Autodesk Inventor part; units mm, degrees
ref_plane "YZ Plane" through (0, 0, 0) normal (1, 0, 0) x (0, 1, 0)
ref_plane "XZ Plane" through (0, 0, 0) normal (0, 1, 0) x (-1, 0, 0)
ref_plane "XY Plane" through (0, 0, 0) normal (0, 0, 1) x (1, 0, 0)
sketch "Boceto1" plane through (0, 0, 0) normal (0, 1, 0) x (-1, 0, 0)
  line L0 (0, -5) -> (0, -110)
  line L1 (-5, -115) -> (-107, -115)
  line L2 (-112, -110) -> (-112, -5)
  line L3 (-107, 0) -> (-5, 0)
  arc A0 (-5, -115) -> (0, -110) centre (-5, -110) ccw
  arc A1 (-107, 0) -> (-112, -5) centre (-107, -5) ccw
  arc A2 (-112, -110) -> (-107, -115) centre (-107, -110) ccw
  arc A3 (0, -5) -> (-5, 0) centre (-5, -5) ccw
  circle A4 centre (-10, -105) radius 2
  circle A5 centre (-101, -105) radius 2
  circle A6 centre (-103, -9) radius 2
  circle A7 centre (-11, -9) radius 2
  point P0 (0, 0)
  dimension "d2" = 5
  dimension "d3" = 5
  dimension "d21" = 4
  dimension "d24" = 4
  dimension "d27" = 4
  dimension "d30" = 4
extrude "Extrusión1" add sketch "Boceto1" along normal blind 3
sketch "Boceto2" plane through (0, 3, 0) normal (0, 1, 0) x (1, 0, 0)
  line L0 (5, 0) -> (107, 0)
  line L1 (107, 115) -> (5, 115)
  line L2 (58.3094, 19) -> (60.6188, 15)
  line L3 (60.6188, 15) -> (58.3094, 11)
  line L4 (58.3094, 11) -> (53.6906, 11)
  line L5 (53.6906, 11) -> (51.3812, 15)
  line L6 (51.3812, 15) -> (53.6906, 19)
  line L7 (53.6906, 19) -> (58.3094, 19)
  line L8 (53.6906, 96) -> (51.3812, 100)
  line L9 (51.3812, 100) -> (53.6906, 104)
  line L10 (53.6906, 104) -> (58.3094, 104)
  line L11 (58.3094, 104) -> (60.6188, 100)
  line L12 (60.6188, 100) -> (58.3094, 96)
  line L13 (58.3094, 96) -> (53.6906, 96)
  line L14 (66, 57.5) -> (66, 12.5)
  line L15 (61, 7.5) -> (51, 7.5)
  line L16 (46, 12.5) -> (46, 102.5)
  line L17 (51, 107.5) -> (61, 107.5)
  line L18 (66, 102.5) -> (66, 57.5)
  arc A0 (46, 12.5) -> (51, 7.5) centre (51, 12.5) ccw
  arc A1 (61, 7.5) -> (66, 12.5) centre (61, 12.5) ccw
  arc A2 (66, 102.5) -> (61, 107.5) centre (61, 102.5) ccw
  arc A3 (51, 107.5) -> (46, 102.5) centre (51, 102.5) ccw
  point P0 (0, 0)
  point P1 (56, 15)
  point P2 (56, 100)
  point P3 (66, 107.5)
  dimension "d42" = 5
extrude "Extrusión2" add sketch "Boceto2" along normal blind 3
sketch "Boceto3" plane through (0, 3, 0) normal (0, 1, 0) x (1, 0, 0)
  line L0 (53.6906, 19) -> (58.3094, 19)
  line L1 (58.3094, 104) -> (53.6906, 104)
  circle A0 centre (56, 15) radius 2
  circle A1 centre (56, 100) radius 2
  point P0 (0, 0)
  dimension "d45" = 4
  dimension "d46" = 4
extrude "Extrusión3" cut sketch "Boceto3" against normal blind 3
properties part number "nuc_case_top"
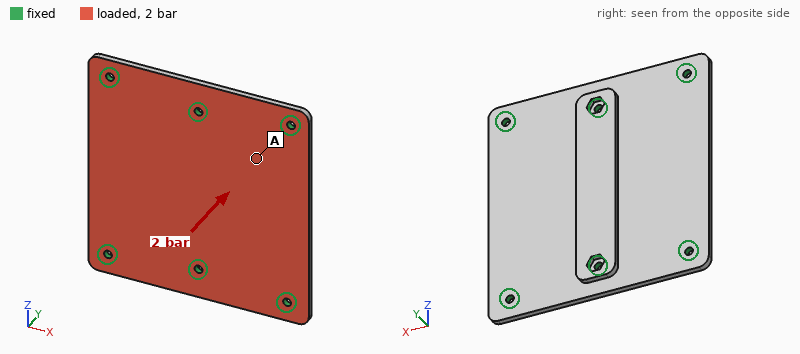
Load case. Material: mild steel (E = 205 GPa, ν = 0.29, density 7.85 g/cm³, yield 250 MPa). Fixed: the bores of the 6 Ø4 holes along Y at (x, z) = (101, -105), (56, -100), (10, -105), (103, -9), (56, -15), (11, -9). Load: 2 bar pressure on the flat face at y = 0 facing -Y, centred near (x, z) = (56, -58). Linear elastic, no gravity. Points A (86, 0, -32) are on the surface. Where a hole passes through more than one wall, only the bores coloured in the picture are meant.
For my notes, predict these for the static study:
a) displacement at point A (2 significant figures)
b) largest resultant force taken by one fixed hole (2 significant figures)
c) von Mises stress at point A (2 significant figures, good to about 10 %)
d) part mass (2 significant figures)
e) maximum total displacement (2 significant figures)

33 µm
890 N
17 MPa
350 g
87 µm
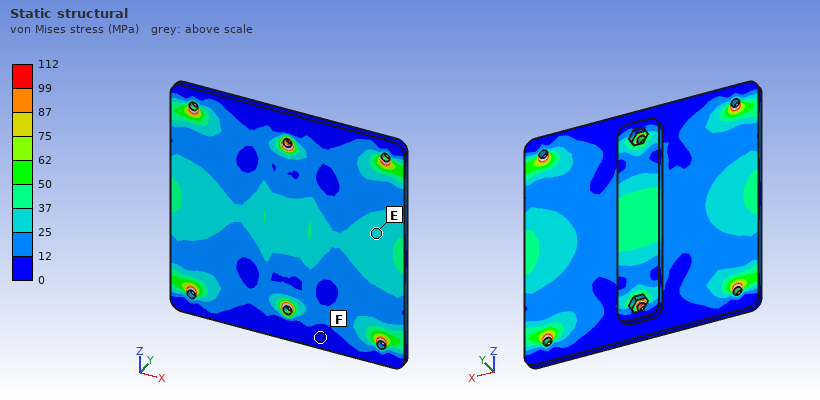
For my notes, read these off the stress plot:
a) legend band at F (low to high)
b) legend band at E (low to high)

0 to 12 MPa
25 to 37 MPa
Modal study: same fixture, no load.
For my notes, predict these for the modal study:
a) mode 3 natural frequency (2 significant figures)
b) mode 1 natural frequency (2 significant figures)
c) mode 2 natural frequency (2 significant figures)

3400 Hz
2000 Hz
2100 Hz
